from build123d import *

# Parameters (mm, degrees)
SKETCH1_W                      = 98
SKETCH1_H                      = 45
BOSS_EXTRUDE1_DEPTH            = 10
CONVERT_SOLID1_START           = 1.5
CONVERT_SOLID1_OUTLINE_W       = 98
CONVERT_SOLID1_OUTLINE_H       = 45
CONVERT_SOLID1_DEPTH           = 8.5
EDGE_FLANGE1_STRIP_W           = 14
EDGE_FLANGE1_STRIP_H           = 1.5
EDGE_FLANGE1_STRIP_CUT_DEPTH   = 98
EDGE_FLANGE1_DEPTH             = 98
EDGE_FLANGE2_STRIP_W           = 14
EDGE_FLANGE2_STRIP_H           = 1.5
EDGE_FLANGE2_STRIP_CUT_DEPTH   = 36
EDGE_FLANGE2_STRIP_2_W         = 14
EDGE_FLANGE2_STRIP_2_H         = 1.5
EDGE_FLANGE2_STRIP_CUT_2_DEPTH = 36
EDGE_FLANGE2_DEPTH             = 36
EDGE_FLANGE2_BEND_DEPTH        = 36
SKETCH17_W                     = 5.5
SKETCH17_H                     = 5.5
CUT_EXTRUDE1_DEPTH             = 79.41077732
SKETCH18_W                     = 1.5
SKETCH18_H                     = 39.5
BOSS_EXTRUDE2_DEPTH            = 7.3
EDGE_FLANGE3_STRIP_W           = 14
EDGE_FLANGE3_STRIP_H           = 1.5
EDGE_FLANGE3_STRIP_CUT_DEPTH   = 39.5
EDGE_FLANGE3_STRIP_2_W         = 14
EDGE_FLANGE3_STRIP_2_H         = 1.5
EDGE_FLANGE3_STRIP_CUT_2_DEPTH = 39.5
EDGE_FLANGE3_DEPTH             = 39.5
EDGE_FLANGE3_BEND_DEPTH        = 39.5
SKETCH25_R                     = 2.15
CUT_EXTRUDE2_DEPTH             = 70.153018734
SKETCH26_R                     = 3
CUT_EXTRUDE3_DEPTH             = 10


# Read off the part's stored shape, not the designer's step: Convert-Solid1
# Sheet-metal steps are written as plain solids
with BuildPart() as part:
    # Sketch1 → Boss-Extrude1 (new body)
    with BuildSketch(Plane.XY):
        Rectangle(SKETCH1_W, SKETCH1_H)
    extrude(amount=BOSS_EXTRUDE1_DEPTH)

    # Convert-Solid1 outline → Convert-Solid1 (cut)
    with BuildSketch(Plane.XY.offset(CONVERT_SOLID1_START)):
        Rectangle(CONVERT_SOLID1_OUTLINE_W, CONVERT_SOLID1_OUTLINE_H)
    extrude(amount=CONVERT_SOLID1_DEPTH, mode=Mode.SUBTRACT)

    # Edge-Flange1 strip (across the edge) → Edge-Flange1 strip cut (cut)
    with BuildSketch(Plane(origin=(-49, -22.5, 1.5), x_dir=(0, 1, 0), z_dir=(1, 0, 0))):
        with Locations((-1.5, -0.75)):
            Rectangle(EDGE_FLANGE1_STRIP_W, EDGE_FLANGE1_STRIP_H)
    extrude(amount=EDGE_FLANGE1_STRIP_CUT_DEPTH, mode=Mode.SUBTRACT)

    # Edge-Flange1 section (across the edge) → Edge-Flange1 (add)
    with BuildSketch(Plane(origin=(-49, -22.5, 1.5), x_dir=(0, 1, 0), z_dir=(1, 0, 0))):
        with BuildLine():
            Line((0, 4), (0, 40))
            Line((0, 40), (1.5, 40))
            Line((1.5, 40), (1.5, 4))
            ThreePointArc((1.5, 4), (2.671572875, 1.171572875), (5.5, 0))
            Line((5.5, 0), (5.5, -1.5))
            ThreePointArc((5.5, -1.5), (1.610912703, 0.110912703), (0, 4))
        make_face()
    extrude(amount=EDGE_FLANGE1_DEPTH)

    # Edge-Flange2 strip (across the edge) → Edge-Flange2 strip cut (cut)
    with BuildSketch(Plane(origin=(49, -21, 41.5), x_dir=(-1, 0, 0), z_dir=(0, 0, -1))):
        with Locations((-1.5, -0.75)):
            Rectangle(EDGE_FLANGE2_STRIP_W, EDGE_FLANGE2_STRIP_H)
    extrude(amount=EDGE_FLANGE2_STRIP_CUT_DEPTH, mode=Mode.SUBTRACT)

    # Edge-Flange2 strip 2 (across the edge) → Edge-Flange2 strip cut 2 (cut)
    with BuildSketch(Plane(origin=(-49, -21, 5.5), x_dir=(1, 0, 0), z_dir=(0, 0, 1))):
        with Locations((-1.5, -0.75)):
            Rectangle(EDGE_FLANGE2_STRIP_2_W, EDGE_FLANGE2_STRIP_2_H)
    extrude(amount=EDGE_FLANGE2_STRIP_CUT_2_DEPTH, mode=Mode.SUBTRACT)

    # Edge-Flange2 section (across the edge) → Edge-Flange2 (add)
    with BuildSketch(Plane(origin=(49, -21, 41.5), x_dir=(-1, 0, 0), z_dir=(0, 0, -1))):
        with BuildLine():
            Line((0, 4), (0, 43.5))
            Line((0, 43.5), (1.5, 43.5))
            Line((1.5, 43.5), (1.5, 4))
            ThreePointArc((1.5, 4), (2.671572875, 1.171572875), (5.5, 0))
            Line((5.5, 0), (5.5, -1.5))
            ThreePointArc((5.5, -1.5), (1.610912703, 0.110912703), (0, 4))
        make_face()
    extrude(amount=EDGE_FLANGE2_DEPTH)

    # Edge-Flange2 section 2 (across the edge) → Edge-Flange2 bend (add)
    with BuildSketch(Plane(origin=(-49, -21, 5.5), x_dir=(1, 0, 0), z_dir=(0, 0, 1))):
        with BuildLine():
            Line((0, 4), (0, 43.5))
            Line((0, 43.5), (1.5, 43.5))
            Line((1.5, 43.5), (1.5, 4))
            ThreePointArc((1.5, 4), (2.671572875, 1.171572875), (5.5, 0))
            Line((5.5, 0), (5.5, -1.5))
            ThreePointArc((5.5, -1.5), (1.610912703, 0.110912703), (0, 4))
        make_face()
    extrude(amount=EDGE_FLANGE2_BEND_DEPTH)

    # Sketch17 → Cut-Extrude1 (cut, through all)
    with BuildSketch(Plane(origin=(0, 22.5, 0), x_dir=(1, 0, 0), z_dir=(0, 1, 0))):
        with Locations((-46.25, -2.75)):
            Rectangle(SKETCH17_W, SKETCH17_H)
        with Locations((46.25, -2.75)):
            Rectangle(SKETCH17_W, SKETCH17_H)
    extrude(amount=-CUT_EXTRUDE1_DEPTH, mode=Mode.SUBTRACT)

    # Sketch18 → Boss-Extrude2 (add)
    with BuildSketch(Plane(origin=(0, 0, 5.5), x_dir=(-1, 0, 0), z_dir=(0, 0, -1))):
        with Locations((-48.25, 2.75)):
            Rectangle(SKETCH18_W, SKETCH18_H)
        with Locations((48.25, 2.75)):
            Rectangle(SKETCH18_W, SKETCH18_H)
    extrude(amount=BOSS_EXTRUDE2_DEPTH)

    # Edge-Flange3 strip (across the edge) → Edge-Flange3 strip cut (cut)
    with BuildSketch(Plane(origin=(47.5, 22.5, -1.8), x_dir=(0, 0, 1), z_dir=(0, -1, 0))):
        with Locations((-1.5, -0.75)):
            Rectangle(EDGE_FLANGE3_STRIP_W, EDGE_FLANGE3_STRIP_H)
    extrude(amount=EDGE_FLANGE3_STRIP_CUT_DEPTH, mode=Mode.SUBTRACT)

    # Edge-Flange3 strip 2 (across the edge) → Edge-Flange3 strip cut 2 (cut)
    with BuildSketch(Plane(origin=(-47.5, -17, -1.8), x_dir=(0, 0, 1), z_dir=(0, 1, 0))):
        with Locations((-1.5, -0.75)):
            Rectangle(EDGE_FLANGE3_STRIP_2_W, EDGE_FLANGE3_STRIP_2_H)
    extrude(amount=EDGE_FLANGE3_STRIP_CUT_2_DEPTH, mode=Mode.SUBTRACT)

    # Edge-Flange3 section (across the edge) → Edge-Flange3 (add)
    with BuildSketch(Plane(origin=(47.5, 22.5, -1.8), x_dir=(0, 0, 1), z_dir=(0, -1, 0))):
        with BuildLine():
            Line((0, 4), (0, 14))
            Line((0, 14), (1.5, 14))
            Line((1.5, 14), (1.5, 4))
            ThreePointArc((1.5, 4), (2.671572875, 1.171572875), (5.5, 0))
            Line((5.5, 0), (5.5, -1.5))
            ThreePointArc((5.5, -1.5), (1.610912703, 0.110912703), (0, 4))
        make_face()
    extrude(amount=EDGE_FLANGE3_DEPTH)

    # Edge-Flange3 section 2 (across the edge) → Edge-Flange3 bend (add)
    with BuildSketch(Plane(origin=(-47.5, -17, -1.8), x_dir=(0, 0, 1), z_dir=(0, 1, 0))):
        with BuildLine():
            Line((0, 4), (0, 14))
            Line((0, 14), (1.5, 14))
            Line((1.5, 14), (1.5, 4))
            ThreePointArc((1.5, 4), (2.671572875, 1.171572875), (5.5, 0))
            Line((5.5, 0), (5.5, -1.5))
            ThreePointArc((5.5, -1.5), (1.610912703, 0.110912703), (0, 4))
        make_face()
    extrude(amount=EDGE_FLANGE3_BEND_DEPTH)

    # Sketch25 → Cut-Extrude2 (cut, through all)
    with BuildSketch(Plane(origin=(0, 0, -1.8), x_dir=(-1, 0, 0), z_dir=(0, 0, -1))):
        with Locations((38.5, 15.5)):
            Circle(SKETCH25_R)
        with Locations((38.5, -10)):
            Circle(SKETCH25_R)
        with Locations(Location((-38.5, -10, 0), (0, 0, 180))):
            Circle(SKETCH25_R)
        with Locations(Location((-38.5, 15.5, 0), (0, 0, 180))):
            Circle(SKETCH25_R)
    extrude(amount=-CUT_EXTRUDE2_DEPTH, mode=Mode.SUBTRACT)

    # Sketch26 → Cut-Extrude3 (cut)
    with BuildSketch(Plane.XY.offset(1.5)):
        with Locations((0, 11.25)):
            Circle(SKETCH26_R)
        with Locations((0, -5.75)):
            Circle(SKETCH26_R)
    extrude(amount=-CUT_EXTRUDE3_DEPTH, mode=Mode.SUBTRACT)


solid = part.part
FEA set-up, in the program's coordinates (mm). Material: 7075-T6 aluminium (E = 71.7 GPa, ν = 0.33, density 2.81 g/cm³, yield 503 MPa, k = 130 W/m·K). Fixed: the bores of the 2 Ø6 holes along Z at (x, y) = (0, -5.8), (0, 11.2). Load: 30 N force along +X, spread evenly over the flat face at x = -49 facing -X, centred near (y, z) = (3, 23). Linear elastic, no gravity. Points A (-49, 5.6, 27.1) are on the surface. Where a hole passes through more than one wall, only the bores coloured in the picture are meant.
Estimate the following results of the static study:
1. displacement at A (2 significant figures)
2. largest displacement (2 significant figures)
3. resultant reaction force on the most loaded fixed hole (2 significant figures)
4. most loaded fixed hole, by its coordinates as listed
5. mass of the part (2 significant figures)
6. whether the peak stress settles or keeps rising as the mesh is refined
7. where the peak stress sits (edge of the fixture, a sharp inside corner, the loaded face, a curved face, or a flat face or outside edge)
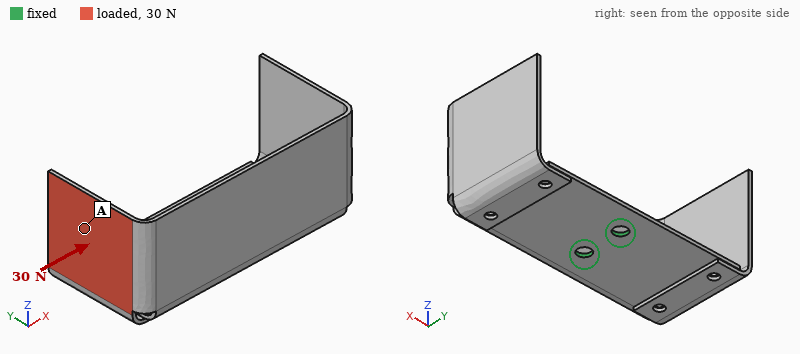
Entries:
0.83 mm
1.4 mm
18 N
(0, 11.2)
50 g
keeps rising
a sharp inside corner
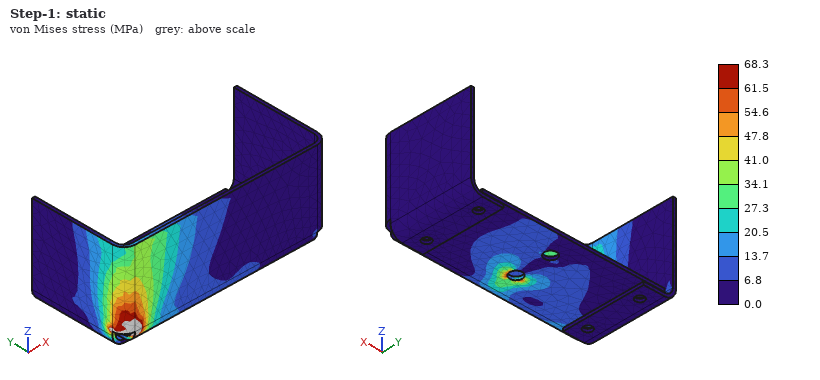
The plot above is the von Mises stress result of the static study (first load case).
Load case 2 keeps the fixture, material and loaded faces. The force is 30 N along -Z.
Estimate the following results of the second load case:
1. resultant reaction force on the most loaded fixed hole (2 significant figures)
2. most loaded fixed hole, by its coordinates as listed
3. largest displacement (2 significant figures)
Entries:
20 N
(0, -5.8)
1.4 mm
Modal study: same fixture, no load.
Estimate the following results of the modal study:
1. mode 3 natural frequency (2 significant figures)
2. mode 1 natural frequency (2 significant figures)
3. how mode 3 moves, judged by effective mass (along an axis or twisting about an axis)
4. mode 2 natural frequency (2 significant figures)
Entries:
260 Hz
220 Hz
along X
240 Hz
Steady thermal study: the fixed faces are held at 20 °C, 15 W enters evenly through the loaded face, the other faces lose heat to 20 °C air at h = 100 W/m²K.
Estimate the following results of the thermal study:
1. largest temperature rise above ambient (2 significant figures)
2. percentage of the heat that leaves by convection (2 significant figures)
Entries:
39 K
93 %
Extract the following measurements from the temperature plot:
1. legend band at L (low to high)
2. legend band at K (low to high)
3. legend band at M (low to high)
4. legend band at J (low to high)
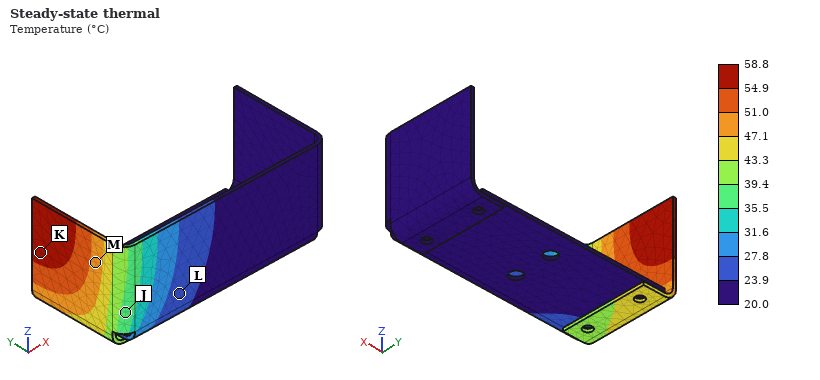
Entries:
23.9 to 27.8 °C
54.9 to 58.8 °C
47.1 to 51.0 °C
35.5 to 39.4 °C
